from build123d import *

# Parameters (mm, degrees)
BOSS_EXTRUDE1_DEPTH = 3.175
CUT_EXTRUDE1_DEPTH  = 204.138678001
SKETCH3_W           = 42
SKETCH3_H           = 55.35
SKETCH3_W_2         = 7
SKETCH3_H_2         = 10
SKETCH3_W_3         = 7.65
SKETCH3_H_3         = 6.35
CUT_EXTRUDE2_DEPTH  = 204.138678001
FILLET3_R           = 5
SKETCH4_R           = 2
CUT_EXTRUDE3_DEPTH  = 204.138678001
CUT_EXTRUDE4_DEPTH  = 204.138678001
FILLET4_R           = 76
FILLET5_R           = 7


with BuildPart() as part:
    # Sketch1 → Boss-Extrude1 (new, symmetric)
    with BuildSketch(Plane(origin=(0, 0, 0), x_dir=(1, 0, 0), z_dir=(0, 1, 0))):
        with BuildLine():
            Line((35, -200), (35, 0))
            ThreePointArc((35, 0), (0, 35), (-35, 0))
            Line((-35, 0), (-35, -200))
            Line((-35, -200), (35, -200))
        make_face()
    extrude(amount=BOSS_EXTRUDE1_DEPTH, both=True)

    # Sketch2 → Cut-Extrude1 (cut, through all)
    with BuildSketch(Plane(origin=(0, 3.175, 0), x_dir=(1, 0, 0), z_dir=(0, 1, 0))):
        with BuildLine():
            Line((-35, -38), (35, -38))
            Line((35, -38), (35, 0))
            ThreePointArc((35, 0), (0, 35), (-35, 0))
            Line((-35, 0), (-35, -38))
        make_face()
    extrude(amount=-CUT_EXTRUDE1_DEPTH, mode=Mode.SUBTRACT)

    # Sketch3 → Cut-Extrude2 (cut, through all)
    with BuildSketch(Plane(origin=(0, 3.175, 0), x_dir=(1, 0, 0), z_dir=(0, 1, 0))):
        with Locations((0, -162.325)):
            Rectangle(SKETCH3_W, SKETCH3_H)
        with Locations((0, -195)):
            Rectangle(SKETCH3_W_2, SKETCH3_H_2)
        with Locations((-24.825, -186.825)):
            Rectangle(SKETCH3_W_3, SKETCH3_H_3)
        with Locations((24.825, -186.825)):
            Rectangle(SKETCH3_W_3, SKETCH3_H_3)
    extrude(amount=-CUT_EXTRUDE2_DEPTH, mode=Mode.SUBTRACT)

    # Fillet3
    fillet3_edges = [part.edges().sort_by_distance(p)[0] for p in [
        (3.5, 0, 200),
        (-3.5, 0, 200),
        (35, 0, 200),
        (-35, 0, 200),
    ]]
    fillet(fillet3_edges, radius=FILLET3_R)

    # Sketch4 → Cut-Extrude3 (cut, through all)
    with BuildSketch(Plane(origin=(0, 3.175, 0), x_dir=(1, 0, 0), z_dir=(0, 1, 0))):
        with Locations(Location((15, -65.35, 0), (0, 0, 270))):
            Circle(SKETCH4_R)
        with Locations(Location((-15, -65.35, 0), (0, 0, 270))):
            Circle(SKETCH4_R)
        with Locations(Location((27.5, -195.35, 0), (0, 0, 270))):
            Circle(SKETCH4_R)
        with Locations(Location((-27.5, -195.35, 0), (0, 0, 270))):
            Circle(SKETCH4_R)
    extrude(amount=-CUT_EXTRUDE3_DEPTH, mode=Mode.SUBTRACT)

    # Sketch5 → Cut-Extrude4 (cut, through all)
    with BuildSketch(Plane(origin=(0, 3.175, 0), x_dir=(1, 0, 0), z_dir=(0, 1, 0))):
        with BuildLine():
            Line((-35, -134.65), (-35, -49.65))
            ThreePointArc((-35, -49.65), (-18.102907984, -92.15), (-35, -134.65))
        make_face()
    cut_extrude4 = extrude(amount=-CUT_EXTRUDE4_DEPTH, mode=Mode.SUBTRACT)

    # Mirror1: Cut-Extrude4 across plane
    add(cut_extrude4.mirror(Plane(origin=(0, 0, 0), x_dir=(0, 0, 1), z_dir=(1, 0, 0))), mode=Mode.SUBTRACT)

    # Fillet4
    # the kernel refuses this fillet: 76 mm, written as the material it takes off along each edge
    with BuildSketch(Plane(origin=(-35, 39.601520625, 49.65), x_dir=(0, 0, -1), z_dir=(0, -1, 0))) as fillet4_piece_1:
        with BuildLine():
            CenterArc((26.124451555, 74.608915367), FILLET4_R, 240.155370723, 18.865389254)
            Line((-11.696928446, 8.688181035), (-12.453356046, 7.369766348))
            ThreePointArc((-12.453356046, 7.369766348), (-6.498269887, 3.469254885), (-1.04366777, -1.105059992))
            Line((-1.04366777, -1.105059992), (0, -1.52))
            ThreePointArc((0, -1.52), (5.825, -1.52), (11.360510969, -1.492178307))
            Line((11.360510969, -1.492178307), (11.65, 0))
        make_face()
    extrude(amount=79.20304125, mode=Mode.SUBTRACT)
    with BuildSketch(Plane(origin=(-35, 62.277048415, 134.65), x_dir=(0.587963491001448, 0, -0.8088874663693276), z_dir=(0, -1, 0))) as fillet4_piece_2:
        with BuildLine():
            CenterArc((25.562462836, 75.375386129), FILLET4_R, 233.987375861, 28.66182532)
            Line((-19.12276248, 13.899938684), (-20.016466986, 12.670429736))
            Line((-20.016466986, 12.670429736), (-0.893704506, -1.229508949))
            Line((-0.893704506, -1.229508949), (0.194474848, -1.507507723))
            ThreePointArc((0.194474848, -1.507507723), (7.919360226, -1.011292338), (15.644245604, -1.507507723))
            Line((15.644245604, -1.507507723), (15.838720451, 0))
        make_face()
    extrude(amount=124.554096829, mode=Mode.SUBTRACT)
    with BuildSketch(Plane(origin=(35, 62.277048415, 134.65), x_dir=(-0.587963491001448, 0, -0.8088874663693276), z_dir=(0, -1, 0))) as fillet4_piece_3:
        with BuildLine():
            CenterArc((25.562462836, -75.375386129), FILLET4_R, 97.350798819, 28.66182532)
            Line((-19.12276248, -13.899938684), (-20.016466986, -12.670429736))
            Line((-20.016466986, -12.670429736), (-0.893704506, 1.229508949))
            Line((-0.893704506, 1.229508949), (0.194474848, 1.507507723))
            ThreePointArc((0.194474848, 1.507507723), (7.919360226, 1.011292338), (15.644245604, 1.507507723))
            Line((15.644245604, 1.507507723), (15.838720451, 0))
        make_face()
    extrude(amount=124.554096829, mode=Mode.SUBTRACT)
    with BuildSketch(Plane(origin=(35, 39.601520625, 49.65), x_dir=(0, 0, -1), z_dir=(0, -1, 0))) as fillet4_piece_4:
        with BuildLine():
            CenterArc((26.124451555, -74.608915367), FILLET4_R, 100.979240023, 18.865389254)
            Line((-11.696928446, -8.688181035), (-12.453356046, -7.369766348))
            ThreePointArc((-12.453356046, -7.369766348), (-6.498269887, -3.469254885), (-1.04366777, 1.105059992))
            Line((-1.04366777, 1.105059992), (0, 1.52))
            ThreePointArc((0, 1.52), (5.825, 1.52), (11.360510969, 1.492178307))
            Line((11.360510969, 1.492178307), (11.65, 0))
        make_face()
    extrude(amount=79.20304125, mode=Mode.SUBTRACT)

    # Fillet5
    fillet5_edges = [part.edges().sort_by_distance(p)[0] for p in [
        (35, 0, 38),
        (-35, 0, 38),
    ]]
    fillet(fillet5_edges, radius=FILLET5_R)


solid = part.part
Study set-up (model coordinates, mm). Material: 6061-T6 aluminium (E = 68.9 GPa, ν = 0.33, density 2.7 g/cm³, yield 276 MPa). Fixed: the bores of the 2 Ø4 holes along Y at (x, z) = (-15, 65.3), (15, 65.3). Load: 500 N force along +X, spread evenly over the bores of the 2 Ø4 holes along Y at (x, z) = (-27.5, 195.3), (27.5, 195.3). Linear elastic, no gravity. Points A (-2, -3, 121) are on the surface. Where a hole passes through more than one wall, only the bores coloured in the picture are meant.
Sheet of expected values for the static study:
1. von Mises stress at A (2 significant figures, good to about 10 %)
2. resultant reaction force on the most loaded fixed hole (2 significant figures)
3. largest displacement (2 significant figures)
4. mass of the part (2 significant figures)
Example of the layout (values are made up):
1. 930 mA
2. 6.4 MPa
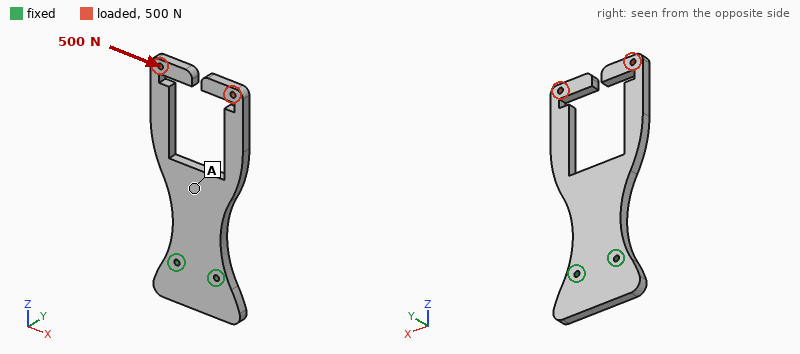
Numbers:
1. 21 MPa
2. 2.1 kN
3. 0.80 mm
4. 110 g
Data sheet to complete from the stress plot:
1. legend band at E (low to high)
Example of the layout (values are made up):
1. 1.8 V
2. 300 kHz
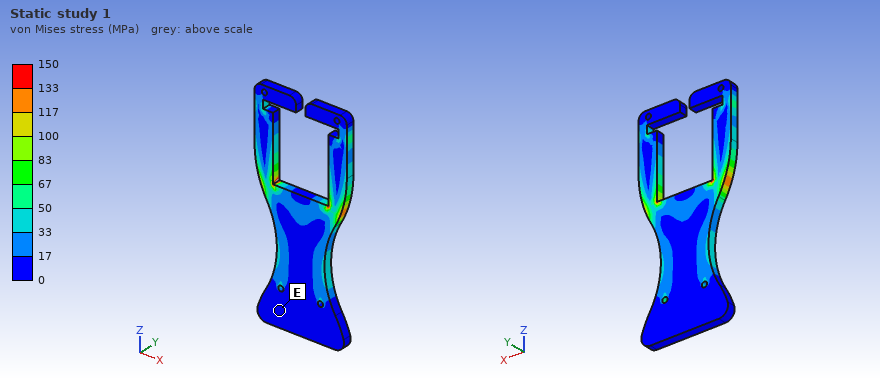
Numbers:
1. 0 to 17 MPa
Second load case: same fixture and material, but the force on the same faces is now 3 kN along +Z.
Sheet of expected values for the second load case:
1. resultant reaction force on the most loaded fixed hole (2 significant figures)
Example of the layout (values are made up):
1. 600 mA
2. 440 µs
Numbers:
1. 1.5 kN
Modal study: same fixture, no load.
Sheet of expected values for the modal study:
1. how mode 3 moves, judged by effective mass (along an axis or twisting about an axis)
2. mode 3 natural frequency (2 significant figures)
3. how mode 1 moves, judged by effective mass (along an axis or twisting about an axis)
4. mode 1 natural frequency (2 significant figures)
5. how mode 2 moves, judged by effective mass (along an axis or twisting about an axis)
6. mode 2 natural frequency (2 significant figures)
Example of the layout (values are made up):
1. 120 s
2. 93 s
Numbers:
1. along X
2. 1000 Hz
3. along Y
4. 290 Hz
5. twisting about Z
6. 540 Hz
